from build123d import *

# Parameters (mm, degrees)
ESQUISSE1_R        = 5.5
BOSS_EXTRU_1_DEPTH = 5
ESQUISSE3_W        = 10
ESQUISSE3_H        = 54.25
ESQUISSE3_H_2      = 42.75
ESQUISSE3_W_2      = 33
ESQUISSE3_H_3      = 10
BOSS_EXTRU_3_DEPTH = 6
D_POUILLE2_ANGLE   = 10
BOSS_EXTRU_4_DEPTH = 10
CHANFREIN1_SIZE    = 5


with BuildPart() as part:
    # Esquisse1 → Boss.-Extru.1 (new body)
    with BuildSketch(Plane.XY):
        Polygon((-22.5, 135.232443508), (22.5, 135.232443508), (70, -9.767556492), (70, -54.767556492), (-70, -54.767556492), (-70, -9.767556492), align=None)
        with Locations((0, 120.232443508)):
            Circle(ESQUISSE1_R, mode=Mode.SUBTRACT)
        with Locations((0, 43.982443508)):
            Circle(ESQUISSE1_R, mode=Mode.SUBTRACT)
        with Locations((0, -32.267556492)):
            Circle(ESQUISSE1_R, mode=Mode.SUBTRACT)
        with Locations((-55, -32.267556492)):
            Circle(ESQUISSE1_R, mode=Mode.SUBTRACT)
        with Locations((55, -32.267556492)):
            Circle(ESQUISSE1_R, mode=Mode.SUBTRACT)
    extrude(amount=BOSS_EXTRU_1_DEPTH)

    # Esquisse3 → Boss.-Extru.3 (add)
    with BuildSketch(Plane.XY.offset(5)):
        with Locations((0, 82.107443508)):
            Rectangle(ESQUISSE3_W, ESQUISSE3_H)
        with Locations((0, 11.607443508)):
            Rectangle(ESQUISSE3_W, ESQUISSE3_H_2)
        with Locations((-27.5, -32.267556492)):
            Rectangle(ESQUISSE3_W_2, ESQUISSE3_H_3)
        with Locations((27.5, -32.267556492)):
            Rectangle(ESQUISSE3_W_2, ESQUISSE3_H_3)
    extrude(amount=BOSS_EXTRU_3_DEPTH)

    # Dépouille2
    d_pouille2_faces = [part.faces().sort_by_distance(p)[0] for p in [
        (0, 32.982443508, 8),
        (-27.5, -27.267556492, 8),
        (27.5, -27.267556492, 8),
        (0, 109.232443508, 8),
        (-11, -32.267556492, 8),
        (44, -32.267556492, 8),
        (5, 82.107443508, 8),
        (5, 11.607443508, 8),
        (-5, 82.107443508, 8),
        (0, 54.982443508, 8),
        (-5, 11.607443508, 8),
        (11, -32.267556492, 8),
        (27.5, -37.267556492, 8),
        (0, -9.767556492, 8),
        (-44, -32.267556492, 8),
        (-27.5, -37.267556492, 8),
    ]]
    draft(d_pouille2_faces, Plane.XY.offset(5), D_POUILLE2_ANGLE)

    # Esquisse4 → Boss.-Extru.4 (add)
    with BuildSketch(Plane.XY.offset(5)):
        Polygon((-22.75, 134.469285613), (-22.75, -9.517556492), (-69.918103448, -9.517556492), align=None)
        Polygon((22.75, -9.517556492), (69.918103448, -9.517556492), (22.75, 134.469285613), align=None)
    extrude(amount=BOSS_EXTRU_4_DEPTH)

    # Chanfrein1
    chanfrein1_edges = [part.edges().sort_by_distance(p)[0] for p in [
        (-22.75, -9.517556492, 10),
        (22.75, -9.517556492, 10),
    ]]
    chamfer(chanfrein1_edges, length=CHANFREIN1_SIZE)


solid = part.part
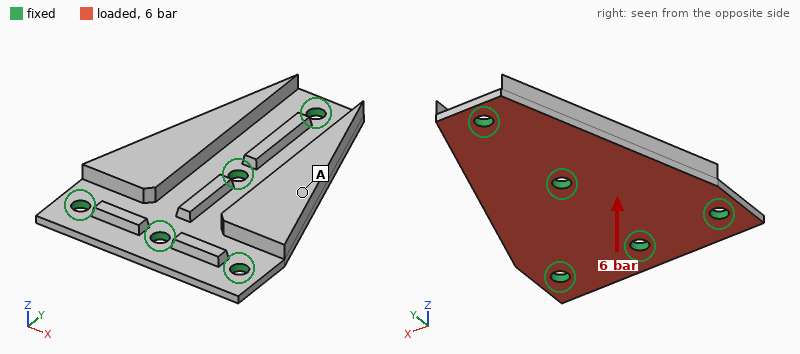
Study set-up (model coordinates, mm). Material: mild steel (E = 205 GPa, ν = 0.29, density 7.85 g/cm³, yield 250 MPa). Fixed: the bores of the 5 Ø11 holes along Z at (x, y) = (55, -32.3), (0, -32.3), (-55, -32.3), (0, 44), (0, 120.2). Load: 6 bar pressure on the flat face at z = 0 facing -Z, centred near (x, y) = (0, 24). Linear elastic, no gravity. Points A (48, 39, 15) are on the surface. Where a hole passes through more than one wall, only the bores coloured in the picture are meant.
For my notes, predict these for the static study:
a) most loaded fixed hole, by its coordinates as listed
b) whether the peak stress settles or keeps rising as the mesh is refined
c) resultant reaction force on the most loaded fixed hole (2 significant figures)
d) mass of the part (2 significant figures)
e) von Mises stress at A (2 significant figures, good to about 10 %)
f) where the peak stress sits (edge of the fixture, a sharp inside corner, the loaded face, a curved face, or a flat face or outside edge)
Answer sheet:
(0, 44)
keeps rising
3.7 kN
1.4 kg
16 MPa
edge of the fixture
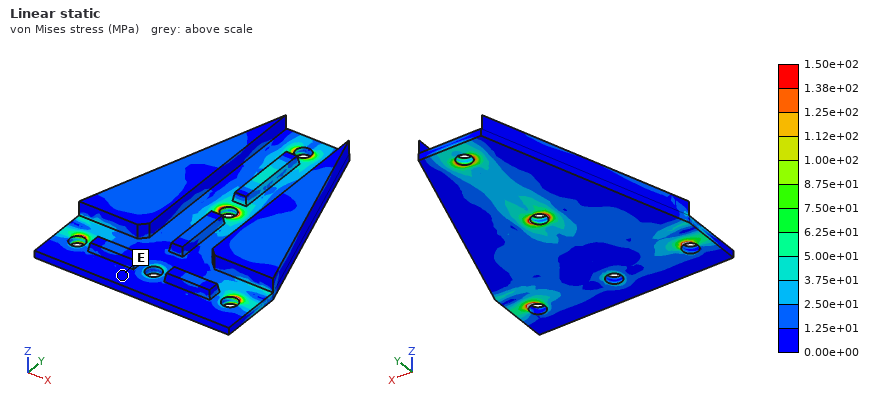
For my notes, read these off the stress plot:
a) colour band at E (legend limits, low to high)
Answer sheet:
0.00e+00 to 1.25e+01 MPa
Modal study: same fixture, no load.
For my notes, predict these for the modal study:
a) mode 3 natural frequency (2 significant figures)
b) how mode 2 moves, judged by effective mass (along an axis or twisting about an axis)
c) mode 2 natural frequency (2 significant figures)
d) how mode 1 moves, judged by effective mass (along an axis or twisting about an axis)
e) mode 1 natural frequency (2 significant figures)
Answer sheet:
4400 Hz
along Z
2200 Hz
twisting about Y
2000 Hz
